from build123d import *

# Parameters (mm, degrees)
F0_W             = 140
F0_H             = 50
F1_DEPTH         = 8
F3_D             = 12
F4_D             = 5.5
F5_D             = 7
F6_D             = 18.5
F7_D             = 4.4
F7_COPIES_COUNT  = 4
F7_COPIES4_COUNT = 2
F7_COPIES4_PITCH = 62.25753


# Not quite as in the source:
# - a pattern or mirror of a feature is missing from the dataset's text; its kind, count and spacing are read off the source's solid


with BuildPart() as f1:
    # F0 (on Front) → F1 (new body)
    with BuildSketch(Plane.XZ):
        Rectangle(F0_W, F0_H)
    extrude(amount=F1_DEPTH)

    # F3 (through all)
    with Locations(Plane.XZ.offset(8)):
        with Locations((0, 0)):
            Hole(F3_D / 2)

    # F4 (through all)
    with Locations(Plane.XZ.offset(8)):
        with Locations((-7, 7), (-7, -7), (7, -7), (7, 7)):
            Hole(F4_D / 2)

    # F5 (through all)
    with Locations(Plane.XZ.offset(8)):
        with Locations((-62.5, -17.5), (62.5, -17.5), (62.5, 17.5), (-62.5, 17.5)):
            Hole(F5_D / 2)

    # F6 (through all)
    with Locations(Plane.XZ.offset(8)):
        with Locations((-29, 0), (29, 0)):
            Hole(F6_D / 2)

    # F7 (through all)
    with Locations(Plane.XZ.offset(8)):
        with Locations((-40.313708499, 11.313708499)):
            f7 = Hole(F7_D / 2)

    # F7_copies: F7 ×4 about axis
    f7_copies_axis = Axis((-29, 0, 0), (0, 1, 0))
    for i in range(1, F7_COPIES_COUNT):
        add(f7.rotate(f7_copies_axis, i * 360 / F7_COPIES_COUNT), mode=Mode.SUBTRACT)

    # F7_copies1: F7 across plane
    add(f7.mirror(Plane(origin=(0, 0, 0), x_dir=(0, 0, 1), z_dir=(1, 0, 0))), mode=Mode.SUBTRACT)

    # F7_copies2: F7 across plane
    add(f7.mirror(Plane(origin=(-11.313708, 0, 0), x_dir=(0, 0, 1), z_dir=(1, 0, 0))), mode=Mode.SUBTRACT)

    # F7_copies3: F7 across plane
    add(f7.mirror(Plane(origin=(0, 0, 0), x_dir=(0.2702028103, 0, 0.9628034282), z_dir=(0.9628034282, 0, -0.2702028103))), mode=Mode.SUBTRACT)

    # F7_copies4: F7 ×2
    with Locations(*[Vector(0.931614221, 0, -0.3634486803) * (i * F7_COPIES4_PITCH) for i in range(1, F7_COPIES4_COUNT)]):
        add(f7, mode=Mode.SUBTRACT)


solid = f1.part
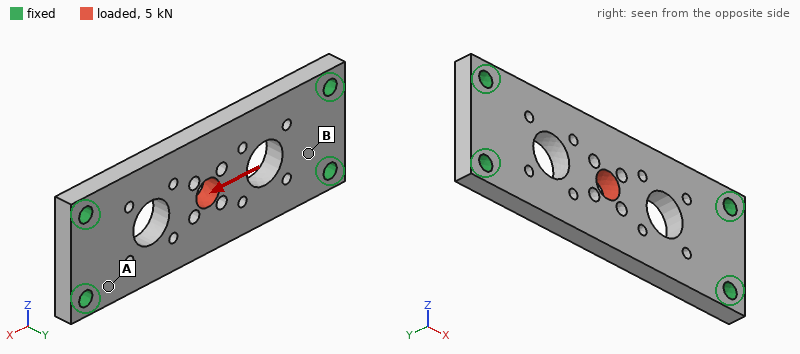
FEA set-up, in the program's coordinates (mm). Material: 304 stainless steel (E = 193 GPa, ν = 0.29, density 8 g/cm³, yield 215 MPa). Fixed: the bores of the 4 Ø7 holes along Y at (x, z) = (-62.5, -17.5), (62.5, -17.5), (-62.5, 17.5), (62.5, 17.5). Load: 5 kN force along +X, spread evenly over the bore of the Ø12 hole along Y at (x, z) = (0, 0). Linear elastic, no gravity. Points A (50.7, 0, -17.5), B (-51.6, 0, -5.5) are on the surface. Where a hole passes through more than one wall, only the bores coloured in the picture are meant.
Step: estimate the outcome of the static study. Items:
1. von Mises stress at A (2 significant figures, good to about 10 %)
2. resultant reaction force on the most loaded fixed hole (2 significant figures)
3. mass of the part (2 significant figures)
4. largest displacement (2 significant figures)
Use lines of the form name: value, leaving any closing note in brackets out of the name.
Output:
von Mises stress at A: 11 MPa
resultant reaction force on the most loaded fixed hole: 1.3 kN
mass of the part: 380 g
largest displacement: 5.3 µm
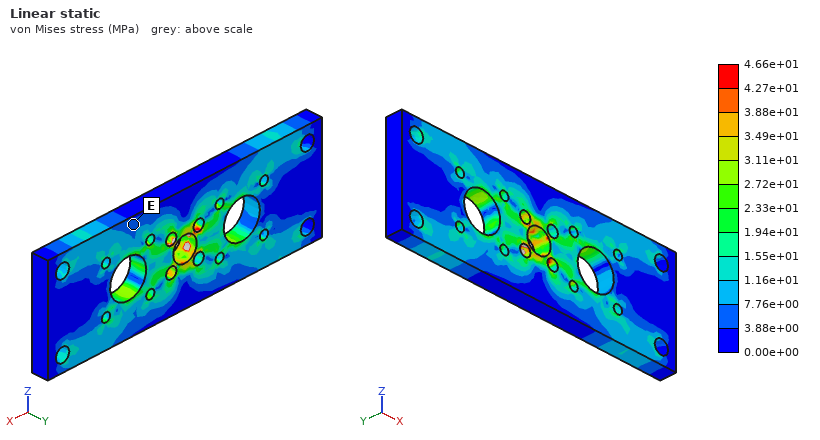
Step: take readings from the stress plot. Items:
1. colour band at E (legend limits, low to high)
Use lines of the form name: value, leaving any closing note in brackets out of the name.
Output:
colour band at E: 3.88e+00 to 7.76e+00 MPa
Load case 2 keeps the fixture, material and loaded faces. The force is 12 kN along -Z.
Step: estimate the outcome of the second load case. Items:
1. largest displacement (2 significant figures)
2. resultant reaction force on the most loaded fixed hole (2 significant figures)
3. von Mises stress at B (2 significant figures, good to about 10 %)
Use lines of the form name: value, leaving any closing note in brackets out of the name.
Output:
largest displacement: 35 µm
resultant reaction force on the most loaded fixed hole: 5.6 kN
von Mises stress at B: 43 MPa
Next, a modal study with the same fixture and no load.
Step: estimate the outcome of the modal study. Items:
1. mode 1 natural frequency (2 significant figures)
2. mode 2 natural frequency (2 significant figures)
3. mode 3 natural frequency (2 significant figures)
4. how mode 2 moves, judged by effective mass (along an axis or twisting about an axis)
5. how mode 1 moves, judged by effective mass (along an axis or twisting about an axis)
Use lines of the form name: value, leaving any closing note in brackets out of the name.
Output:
mode 1 natural frequency: 2600 Hz
mode 2 natural frequency: 4300 Hz
mode 3 natural frequency: 6800 Hz
how mode 2 moves, judged by effective mass: twisting about X
how mode 1 moves, judged by effective mass: along Y
